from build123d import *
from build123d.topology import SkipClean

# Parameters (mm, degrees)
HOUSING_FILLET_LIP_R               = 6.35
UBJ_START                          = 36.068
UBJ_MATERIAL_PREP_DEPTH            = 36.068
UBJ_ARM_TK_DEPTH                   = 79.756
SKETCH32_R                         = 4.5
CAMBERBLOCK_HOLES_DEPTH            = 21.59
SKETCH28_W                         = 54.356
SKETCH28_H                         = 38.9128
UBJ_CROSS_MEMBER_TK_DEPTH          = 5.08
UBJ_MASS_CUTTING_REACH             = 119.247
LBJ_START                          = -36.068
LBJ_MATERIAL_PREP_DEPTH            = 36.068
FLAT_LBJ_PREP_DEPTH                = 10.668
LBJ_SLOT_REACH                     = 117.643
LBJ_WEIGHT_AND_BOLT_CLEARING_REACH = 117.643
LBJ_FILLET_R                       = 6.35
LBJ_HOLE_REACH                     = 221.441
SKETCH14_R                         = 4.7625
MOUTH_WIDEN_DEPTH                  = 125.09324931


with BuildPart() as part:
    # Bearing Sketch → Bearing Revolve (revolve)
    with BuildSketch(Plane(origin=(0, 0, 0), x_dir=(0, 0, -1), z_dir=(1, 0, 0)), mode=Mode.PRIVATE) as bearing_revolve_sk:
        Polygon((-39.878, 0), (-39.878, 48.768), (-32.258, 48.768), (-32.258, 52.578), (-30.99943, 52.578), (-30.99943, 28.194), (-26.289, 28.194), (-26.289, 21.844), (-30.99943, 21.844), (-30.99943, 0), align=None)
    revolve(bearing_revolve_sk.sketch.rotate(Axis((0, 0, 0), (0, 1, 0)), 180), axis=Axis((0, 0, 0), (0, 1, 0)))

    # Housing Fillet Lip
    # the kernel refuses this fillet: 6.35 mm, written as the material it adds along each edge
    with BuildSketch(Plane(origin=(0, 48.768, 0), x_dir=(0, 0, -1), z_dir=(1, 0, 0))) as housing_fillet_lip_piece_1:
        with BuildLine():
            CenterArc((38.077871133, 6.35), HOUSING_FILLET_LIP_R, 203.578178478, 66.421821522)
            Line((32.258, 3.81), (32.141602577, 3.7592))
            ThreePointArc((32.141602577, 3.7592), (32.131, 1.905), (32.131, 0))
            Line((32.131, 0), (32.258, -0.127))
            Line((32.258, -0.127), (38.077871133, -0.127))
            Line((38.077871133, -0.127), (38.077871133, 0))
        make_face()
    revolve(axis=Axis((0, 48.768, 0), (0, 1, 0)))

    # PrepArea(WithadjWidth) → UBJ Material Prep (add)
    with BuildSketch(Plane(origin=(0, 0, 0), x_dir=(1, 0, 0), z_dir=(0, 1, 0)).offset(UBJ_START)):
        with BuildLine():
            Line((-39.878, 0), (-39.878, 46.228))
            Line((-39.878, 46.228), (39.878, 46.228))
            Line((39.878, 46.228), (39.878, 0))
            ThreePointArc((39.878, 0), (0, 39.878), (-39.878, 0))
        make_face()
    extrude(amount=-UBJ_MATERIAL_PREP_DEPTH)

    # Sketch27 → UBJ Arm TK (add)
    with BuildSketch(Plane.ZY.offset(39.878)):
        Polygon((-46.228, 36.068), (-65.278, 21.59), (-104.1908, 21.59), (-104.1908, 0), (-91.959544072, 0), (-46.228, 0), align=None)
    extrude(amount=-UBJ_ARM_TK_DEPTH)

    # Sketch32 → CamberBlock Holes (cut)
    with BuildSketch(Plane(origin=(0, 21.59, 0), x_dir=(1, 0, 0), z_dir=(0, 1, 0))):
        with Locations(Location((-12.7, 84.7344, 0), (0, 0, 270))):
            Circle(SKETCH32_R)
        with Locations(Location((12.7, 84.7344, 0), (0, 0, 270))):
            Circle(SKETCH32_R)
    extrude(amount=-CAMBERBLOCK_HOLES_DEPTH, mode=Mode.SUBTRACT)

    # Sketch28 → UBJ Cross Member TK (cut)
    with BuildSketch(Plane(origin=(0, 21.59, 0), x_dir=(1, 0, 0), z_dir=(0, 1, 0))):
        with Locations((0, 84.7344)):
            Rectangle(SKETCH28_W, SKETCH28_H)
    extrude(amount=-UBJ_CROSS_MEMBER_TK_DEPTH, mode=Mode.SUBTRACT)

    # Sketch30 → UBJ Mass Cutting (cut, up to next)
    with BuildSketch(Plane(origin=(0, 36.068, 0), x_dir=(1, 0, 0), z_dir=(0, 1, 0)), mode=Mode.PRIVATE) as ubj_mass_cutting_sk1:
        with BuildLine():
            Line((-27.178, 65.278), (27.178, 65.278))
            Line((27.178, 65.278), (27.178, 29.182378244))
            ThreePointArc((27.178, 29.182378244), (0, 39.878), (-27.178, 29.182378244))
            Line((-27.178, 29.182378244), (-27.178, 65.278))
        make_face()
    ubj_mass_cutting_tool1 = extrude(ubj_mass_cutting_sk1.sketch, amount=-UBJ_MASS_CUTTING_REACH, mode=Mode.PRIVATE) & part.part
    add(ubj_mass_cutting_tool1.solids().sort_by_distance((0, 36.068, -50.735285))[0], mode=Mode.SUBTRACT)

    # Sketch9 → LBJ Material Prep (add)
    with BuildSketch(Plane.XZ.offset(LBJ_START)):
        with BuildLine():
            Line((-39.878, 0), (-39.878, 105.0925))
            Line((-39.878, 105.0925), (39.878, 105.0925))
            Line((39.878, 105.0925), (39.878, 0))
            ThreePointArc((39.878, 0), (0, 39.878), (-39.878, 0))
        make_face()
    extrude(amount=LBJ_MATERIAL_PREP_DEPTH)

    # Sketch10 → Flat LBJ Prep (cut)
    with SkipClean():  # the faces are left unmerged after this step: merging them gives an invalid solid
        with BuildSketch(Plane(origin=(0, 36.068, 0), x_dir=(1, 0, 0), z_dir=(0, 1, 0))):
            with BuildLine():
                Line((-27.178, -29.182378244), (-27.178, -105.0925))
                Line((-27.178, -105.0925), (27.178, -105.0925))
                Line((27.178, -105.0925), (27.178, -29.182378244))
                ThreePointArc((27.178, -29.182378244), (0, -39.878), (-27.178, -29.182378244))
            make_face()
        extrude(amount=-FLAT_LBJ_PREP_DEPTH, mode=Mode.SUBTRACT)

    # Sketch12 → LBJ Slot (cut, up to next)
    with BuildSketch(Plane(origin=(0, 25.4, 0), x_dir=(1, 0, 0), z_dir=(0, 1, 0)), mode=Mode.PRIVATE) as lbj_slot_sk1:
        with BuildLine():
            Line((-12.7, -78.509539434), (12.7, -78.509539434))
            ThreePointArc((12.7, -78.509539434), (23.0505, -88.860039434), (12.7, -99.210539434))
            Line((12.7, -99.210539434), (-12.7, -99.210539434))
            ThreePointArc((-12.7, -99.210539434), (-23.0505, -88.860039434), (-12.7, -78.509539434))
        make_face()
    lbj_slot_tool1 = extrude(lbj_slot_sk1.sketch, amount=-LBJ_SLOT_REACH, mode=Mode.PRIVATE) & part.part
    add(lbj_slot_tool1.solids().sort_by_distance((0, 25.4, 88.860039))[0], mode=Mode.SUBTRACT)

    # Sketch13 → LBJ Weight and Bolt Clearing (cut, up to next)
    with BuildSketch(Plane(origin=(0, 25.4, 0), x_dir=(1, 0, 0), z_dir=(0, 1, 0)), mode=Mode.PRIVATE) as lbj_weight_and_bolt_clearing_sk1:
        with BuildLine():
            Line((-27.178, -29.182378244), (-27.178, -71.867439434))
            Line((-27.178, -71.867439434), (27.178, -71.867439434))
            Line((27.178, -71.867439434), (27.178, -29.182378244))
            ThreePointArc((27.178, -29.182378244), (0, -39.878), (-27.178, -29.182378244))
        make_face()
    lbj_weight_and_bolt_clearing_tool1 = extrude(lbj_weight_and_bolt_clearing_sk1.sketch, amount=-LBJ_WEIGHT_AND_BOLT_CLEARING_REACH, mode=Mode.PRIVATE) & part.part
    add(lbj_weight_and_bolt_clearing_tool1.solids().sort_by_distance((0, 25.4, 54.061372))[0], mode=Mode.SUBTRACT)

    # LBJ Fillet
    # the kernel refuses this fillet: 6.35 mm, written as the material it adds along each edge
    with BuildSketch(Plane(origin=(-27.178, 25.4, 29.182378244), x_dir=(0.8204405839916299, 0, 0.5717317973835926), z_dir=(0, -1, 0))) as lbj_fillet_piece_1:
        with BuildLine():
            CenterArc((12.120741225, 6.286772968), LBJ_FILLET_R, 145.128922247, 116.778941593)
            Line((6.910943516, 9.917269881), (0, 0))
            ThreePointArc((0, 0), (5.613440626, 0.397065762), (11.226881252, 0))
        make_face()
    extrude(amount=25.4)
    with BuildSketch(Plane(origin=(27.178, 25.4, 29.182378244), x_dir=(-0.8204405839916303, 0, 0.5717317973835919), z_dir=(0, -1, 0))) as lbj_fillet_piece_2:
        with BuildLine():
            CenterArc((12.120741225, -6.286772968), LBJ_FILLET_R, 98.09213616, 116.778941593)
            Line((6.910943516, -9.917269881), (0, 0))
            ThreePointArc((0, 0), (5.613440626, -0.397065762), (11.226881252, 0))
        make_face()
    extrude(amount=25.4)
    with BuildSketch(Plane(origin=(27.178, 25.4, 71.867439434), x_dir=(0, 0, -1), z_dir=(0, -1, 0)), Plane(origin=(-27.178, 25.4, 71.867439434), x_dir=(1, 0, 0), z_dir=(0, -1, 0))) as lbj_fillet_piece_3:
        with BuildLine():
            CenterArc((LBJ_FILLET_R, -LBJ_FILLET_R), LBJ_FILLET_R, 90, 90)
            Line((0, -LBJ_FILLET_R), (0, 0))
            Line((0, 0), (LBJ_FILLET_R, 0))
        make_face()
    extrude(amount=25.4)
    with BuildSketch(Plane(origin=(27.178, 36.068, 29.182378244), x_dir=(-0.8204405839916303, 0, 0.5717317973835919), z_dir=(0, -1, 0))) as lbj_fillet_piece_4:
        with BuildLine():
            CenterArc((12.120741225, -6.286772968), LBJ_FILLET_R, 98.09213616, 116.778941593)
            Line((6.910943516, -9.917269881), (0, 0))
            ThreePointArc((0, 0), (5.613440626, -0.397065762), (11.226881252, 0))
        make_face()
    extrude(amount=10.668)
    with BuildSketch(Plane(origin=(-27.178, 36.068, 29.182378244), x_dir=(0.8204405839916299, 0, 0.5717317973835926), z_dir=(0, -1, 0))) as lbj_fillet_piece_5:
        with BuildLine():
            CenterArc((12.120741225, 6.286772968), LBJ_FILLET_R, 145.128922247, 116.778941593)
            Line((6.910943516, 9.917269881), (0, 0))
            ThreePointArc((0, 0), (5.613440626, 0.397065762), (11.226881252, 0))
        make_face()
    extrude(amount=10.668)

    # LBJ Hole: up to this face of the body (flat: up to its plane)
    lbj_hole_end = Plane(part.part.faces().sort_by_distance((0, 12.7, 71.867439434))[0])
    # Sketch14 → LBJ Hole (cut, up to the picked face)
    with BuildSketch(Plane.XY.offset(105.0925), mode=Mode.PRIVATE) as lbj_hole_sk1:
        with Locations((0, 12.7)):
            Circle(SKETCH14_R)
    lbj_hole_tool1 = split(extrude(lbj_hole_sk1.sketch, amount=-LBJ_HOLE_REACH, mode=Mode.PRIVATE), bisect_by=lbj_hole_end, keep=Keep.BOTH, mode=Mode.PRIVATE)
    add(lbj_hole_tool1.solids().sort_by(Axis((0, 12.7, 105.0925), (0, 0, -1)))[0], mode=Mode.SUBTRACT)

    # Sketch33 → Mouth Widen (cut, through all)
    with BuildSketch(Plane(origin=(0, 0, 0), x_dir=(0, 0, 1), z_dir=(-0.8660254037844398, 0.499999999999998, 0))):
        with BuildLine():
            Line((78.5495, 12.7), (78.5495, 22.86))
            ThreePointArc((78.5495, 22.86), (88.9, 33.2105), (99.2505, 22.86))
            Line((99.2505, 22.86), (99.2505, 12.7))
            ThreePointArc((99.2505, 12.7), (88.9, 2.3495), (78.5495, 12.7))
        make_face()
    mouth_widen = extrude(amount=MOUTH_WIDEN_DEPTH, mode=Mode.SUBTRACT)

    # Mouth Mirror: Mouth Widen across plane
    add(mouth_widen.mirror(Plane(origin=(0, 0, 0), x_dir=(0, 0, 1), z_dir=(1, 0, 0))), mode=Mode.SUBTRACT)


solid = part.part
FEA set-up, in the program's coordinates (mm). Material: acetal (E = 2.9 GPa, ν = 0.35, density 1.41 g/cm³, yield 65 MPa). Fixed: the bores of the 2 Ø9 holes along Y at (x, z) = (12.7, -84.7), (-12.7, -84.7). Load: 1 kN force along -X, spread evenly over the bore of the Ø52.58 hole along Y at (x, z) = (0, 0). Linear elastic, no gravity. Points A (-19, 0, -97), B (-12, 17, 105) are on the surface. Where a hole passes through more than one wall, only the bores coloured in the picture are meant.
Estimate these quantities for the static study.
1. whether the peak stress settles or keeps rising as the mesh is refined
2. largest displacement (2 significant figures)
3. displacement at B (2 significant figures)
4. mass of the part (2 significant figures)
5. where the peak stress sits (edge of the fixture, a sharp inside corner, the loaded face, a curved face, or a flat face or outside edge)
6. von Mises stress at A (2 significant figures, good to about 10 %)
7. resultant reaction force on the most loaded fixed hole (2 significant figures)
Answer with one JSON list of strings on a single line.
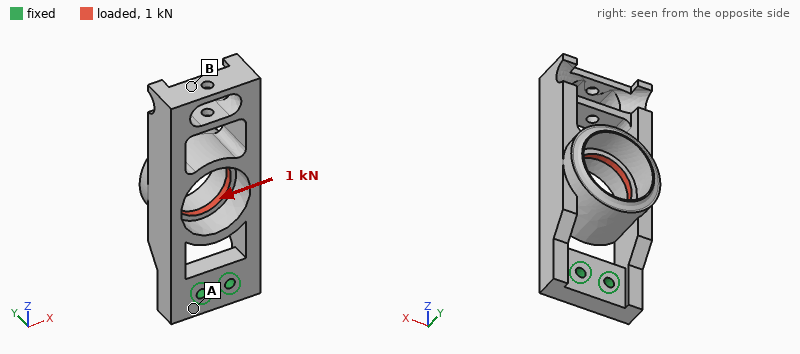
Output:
["keeps rising", "2.2 mm", "2.1 mm", "410 g", "edge of the fixture", "4.9 MPa", "2.3 kN"]
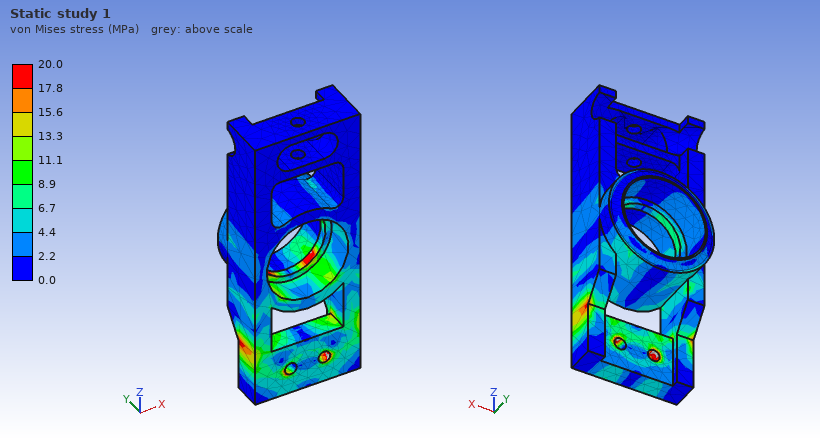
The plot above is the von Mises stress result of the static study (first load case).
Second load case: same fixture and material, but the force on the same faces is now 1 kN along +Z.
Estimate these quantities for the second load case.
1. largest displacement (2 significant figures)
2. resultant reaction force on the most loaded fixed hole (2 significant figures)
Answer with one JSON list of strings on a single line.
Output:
["1.7 mm", "500 N"]
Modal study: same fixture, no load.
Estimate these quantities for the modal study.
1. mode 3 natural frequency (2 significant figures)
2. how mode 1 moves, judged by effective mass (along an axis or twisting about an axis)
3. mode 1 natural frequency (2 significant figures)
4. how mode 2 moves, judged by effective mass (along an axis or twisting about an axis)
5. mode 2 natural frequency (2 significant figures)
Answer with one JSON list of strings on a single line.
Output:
["320 Hz", "along Y", "100 Hz", "along X", "190 Hz"]
